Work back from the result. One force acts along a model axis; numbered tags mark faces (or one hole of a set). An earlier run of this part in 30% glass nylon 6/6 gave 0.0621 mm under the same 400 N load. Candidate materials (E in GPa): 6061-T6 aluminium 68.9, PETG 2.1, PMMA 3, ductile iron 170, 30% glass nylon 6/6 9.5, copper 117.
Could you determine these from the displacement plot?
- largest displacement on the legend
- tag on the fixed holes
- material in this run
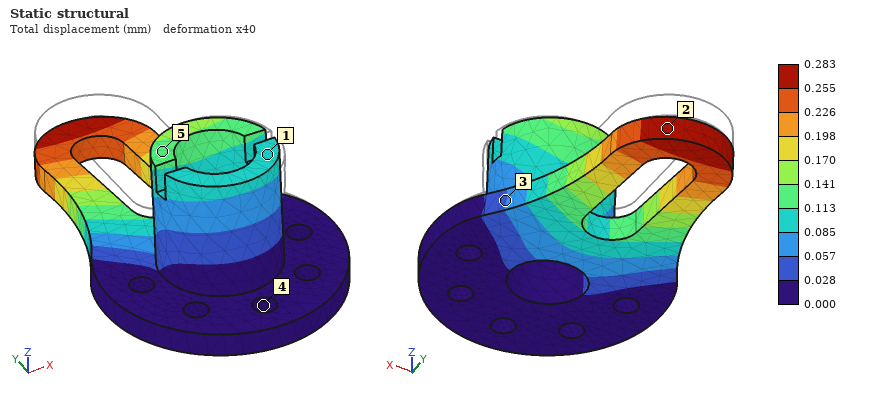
0.283 mm
4
PETG
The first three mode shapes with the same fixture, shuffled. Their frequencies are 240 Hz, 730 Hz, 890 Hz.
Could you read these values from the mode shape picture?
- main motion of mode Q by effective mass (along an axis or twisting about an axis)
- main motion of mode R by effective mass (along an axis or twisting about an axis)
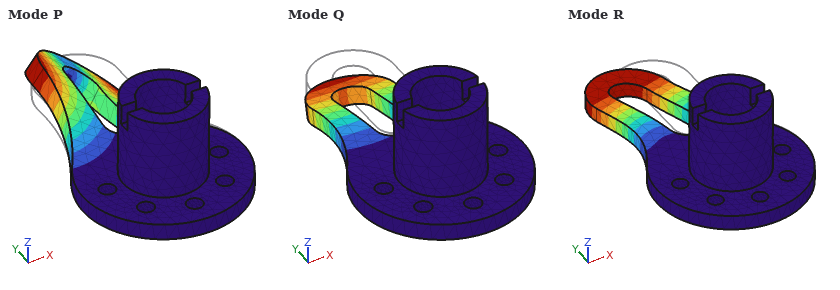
along Z
along X
